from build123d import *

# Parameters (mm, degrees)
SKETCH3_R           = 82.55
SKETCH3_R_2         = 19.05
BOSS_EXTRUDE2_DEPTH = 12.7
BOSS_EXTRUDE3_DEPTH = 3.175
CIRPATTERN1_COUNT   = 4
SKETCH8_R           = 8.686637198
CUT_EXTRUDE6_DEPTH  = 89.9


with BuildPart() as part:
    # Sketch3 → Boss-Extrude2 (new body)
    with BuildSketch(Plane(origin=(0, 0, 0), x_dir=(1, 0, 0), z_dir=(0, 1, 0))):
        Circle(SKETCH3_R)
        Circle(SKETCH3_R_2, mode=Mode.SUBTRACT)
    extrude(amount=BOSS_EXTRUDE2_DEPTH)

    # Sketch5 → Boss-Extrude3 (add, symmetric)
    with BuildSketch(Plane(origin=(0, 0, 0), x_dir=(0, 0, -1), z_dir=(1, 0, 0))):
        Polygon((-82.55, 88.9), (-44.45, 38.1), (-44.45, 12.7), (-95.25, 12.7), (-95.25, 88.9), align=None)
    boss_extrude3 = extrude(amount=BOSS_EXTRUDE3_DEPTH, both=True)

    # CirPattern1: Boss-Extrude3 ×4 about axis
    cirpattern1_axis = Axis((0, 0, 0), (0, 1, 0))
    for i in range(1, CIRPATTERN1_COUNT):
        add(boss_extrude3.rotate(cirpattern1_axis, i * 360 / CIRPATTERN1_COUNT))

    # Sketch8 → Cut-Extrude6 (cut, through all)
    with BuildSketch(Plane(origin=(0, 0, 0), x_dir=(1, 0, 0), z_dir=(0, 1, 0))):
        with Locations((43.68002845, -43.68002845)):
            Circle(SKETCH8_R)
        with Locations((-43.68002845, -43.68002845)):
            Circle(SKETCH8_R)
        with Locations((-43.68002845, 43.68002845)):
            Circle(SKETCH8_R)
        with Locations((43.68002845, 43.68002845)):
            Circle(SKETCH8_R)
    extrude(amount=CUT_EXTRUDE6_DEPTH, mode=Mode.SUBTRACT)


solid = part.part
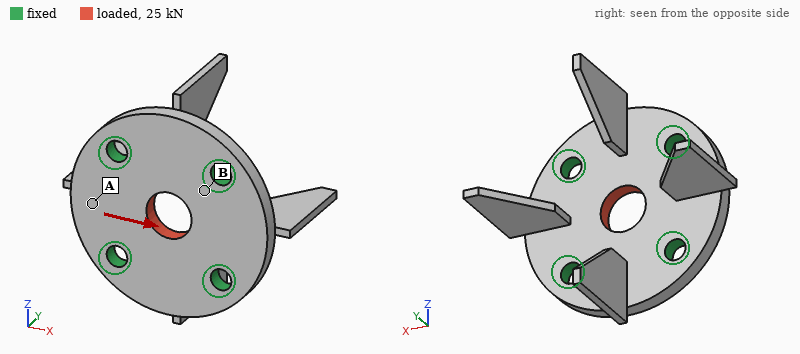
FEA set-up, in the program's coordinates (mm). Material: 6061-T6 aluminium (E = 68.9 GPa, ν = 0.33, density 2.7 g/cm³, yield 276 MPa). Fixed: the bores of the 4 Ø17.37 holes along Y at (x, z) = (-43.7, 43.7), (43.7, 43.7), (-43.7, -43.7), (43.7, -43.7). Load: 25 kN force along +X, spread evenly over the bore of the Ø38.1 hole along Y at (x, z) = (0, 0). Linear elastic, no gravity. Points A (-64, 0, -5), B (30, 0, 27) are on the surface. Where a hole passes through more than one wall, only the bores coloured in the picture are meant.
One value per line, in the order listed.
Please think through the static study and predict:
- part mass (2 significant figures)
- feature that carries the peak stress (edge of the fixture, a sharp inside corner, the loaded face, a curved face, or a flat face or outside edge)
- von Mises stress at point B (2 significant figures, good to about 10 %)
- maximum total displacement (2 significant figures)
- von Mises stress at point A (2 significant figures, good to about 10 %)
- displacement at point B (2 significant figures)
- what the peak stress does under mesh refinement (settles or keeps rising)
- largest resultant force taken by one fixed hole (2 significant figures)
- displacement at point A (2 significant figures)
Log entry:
860 g
edge of the fixture
16 MPa
12 µm
5.1 MPa
4.2 µm
keeps rising
6.5 kN
6.2 µm
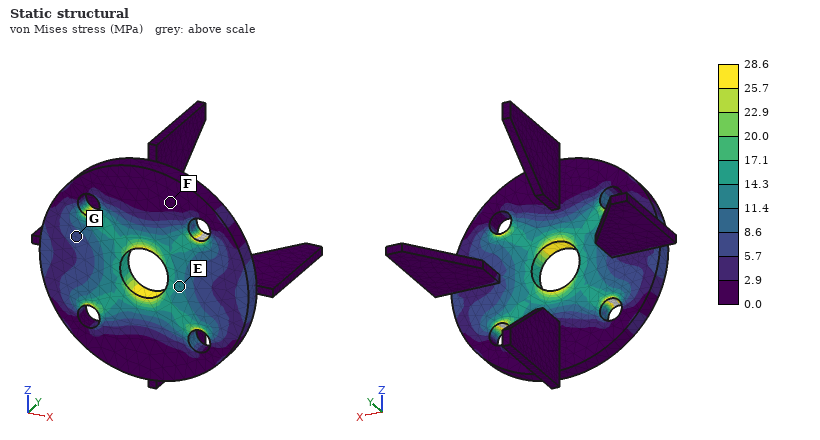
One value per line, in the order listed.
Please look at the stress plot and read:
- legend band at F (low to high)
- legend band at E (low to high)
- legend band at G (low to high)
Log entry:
0.0 to 2.9 MPa
11.4 to 14.3 MPa
5.7 to 8.6 MPa
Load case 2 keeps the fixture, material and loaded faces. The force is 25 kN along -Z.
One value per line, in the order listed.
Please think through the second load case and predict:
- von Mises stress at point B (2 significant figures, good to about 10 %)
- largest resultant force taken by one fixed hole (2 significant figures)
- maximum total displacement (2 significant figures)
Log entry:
15 MPa
6.5 kN
12 µm
